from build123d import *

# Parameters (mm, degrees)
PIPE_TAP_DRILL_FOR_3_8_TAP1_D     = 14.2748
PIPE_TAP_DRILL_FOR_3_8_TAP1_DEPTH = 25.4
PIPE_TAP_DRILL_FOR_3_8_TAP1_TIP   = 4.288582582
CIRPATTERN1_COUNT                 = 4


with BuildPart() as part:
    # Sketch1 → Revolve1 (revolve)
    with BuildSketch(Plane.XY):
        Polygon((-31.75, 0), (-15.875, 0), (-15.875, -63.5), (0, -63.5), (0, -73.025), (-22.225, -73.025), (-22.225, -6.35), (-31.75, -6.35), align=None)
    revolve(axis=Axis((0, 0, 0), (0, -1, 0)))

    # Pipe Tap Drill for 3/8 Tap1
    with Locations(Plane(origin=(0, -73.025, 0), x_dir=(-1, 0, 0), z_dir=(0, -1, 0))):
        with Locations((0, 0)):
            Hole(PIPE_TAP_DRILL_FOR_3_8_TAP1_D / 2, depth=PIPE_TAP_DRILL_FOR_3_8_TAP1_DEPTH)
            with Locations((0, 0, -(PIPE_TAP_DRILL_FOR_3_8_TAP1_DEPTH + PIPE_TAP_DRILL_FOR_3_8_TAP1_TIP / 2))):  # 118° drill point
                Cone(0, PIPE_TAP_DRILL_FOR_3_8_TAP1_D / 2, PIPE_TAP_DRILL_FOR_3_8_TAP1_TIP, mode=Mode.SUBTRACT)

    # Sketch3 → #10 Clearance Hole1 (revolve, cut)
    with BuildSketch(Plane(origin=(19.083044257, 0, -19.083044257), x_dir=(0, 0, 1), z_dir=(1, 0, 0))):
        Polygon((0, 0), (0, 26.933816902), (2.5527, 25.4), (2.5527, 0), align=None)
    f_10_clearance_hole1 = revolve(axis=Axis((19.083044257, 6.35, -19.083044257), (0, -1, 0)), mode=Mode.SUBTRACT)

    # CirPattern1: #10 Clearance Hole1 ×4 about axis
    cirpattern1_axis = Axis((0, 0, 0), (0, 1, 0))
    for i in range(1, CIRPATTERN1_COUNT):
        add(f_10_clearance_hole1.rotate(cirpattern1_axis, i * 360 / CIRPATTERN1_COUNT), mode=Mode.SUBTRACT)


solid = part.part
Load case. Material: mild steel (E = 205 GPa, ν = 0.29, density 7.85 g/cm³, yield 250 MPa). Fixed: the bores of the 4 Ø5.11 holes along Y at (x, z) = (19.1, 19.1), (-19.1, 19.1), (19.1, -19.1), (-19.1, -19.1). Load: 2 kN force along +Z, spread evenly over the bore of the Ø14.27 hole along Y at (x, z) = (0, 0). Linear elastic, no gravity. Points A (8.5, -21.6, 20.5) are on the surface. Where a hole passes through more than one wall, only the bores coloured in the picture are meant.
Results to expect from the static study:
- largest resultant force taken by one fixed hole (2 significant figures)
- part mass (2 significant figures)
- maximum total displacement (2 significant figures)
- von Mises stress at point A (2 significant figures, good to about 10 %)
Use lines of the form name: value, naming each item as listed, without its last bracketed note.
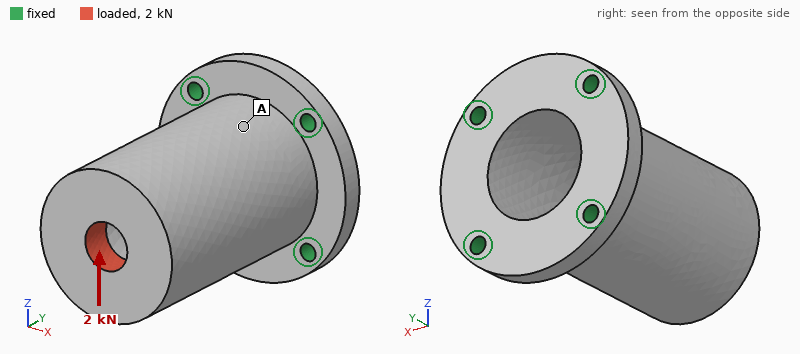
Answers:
largest resultant force taken by one fixed hole: 1.9 kN
part mass: 560 g
maximum total displacement: 22 µm
von Mises stress at point A: 11 MPa
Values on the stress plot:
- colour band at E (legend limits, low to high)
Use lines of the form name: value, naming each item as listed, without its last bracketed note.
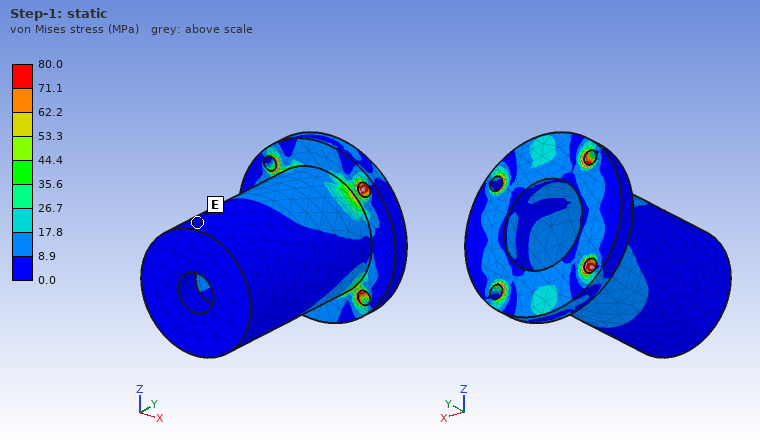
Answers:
colour band at E: 0.0 to 8.9 MPa
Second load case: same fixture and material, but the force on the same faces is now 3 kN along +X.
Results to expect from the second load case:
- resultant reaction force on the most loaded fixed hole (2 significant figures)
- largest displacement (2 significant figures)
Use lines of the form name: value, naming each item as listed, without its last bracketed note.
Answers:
resultant reaction force on the most loaded fixed hole: 2.9 kN
largest displacement: 34 µm
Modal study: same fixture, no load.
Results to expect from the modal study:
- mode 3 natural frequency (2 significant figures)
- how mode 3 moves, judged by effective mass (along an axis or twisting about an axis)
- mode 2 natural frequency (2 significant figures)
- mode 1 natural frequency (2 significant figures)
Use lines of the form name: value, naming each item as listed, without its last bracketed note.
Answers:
mode 3 natural frequency: 9900 Hz
how mode 3 moves, judged by effective mass: along Y
mode 2 natural frequency: 3500 Hz
mode 1 natural frequency: 3500 Hz
